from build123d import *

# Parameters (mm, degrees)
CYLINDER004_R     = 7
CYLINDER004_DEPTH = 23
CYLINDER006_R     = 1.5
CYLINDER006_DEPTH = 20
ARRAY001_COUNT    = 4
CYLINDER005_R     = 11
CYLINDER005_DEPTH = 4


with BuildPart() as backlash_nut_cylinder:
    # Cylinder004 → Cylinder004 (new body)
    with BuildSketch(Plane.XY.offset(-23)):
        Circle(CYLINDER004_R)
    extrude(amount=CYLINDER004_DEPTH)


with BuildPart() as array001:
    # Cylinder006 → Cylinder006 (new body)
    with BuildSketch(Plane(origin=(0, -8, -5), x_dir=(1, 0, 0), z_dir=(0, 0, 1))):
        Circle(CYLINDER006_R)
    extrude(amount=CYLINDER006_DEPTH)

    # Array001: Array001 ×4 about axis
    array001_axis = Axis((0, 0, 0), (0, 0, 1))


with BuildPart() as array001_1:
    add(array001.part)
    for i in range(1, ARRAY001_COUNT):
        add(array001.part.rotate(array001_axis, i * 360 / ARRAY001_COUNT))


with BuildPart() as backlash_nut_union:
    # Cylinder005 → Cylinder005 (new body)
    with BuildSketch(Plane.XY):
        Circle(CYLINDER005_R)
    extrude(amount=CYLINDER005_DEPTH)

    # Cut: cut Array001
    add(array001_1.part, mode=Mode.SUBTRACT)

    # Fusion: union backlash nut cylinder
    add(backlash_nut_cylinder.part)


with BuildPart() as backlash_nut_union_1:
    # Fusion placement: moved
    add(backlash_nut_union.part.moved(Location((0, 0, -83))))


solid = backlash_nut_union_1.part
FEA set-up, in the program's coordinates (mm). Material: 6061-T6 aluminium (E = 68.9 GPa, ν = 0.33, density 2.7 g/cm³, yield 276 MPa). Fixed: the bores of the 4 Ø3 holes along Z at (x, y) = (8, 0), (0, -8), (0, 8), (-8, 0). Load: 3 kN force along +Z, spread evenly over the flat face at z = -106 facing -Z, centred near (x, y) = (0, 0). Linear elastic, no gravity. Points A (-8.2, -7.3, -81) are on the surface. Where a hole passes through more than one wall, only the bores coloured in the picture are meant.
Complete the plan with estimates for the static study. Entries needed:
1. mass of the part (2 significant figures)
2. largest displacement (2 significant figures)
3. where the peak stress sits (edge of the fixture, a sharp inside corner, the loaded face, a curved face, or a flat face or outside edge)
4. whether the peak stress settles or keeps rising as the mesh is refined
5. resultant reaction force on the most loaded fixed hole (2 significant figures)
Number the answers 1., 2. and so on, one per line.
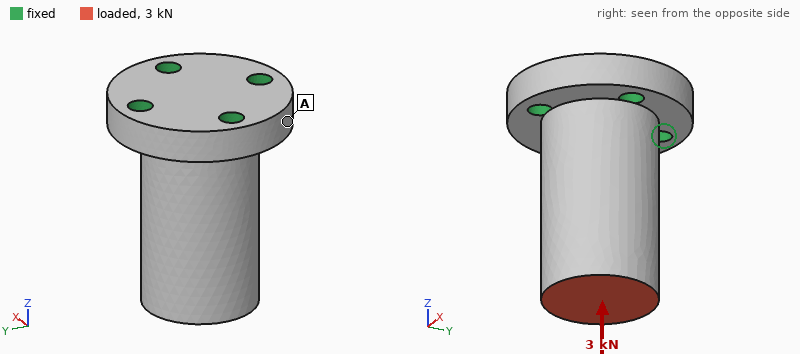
1. 13 g
2. 8.3 µm
3. edge of the fixture
4. keeps rising
5. 790 N
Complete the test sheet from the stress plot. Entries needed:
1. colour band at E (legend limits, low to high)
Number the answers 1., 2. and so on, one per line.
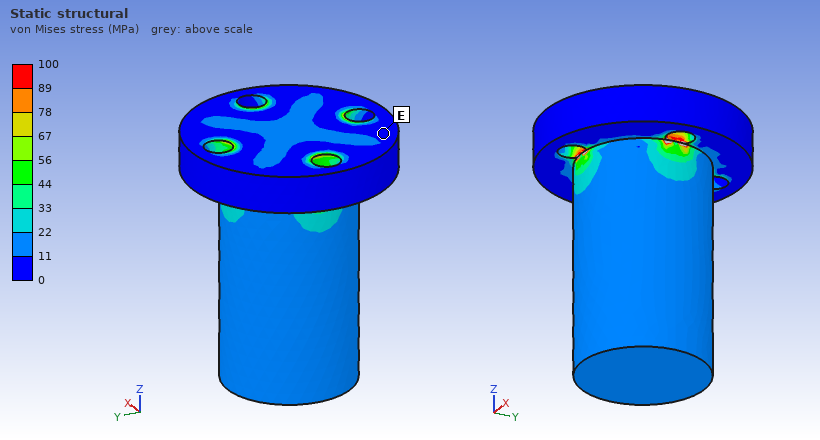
1. 0 to 11 MPa
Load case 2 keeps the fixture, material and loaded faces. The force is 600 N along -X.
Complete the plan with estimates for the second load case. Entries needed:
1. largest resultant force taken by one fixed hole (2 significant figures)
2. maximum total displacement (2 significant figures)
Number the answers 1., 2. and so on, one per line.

1. 990 N
2. 32 µm
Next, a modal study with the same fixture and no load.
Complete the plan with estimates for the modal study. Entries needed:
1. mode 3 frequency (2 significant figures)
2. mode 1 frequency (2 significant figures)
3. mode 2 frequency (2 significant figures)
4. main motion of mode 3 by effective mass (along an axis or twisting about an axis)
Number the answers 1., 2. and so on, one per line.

1. 32 kHz
2. 13 kHz
3. 13 kHz
4. twisting about Z
